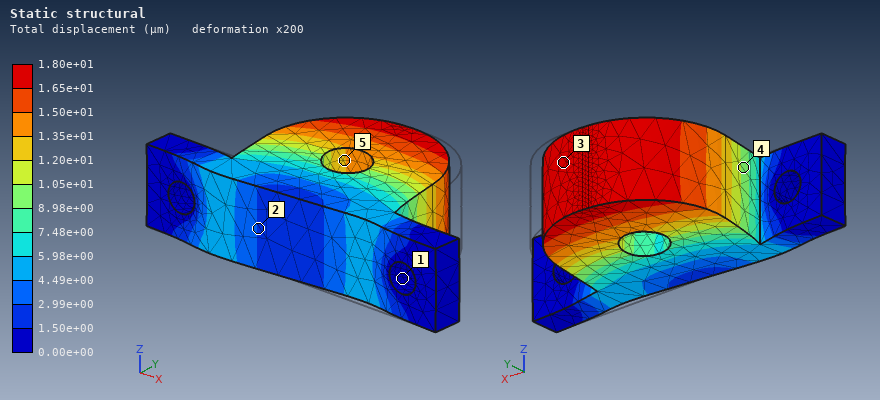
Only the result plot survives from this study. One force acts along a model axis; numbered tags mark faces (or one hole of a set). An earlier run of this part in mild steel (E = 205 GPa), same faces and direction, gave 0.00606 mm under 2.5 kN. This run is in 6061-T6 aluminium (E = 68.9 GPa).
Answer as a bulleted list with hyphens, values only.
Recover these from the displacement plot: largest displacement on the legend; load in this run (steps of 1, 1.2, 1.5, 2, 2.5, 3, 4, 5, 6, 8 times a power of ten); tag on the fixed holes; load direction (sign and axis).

- 1.80e+01 µm
- 2.5 kN
- 1
- -X
